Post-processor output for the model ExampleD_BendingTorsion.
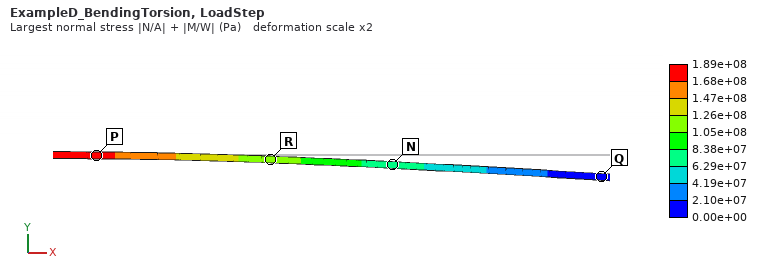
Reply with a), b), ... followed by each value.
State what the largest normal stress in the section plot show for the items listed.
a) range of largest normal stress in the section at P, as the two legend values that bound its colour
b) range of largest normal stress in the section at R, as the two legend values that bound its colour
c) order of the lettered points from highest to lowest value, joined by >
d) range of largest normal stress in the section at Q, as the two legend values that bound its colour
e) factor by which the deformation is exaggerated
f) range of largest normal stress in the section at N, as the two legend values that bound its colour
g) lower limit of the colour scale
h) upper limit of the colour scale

a) 1.68e+08 to 1.89e+08 Pa
b) 1.05e+08 to 1.26e+08 Pa
c) P > R > N > Q
d) 0.00e+00 to 2.10e+07 Pa
e) 2
f) 6.29e+07 to 8.38e+07 Pa
g) 0.00e+00 Pa
h) 1.89e+08 Pa
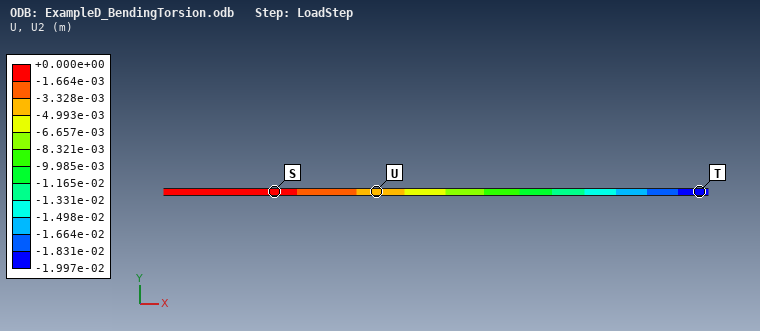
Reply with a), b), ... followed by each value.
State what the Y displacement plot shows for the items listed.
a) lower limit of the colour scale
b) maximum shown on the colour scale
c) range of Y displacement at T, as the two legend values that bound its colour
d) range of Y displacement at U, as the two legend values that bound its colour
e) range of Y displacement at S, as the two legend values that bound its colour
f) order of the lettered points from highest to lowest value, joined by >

a) -1.997e-02 m
b) +0.000e+00 m
c) -1.997e-02 to -1.831e-02 m
d) -4.993e-03 to -3.328e-03 m
e) -1.664e-03 to +0.000e+00 m
f) S > U > T
